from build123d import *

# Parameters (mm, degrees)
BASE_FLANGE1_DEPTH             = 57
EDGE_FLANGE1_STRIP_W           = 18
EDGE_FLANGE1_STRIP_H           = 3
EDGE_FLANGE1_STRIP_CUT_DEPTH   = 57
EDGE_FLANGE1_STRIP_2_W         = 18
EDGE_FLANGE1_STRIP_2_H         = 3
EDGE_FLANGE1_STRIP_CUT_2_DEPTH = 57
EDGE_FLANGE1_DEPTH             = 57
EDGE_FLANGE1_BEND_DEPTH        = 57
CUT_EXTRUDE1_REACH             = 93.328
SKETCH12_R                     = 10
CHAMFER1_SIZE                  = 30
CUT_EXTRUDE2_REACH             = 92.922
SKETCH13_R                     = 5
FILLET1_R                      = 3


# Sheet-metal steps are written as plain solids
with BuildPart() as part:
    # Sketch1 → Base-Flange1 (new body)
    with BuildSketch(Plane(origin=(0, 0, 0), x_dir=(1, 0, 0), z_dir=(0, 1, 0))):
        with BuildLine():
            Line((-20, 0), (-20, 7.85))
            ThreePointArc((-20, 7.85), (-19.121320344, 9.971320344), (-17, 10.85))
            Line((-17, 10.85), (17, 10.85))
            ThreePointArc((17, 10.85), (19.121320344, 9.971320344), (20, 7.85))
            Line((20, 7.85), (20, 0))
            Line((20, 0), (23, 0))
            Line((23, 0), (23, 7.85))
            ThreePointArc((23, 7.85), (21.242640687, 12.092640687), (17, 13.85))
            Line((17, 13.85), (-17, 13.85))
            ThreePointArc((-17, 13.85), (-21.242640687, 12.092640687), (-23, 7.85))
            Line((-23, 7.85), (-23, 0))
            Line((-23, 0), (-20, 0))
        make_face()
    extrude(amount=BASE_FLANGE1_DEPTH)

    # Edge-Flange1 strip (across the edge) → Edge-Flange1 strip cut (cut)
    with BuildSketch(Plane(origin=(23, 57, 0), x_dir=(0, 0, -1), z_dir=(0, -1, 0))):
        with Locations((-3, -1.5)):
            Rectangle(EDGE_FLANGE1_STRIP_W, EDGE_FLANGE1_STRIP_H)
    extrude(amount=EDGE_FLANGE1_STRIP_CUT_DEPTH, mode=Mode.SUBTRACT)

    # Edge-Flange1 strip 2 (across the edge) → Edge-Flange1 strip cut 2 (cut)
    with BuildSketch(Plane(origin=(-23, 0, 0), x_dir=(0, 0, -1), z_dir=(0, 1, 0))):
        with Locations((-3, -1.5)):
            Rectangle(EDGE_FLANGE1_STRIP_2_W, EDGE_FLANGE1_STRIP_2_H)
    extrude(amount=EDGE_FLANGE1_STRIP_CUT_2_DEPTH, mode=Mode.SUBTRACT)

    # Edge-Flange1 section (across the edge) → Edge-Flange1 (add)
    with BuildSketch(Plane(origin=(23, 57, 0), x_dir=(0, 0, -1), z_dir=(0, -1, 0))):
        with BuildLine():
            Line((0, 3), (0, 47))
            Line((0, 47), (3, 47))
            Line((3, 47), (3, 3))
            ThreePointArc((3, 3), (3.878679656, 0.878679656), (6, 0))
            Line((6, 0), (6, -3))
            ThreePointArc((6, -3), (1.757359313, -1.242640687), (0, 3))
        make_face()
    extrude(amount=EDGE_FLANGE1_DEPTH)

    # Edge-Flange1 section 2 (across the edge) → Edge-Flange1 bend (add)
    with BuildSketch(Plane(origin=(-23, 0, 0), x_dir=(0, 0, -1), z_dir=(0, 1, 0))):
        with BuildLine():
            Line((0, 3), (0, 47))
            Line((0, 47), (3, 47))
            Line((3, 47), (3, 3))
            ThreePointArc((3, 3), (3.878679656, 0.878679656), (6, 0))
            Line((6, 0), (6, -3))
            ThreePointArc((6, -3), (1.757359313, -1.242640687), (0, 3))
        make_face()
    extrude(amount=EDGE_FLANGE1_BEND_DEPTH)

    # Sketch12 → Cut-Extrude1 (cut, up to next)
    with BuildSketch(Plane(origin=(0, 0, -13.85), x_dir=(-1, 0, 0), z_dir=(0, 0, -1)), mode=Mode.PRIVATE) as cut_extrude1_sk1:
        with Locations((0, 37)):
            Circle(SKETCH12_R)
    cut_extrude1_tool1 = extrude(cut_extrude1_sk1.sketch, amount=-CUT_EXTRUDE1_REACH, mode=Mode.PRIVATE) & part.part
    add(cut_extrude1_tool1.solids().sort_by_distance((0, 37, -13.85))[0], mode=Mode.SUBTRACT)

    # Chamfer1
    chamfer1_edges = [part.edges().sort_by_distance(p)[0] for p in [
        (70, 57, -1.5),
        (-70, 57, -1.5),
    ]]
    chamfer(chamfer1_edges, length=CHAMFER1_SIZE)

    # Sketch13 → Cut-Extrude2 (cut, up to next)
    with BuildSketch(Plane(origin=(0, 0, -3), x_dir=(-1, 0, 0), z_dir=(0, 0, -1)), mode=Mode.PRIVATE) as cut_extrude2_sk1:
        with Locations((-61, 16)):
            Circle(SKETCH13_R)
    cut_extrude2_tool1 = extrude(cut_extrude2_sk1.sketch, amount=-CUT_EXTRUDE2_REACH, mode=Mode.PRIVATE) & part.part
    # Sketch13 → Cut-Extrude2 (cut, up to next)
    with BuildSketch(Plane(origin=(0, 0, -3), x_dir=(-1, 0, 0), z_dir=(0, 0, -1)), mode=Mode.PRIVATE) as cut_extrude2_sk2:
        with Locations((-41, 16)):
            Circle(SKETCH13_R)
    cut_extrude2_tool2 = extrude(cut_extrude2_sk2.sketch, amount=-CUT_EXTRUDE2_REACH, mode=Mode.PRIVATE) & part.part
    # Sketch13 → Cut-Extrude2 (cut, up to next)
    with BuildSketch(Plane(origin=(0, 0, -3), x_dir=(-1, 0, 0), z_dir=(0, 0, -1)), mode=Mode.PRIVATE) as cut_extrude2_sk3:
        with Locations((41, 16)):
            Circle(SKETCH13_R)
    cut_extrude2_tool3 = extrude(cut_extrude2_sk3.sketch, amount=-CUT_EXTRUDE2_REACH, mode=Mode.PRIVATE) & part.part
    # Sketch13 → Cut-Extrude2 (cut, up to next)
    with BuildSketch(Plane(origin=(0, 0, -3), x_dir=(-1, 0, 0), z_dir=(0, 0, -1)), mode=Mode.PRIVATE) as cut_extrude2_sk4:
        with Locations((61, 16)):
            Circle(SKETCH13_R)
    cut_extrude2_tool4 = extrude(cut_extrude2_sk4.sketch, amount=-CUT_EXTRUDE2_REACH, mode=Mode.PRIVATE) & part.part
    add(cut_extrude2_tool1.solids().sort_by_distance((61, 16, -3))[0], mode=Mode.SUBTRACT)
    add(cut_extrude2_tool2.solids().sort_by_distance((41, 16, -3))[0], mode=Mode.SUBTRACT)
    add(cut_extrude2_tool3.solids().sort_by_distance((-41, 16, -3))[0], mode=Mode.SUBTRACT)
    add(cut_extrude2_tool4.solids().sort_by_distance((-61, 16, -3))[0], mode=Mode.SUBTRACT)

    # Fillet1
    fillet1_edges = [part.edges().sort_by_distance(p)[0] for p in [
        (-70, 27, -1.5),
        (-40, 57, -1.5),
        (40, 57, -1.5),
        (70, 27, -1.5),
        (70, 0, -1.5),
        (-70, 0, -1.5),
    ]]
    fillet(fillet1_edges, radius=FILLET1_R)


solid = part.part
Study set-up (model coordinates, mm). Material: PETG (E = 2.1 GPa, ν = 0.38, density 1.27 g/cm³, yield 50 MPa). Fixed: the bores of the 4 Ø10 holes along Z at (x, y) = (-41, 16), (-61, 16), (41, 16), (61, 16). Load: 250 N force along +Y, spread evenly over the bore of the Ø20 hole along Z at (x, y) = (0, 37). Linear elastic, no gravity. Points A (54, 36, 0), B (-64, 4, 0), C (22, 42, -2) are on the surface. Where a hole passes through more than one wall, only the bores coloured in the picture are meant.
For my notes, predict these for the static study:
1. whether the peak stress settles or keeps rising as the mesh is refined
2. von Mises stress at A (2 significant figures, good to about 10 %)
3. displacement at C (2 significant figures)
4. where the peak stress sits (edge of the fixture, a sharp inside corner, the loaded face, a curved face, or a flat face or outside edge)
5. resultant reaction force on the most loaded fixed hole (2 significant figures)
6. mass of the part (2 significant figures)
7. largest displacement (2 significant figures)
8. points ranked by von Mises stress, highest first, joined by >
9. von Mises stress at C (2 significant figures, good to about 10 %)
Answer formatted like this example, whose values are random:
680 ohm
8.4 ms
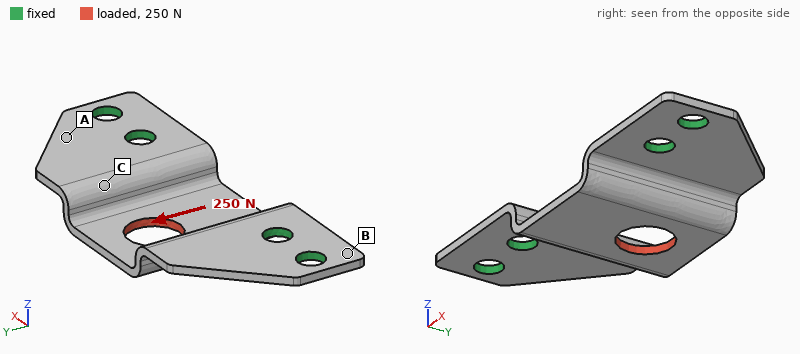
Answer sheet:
keeps rising
7.1 MPa
0.99 mm
edge of the fixture
220 N
28 g
1.7 mm
A > C > B
3.7 MPa
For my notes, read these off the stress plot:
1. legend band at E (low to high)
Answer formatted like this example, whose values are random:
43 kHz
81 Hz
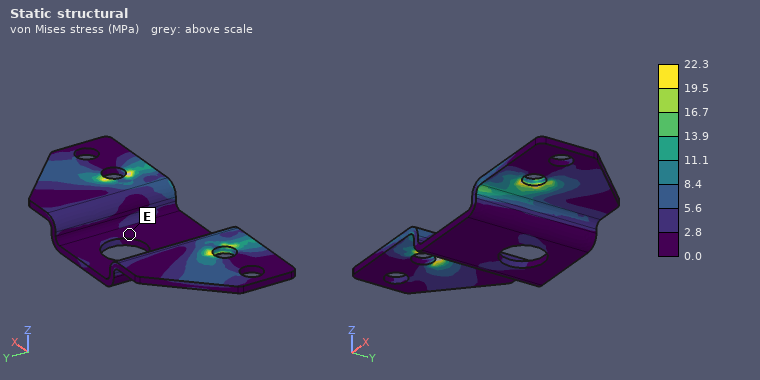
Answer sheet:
0.0 to 2.8 MPa
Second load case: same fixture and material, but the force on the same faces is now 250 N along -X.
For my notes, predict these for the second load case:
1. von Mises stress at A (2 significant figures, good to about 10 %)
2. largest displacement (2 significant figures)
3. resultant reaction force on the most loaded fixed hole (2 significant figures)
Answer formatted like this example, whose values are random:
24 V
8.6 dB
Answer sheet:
1.0 MPa
0.35 mm
100 N
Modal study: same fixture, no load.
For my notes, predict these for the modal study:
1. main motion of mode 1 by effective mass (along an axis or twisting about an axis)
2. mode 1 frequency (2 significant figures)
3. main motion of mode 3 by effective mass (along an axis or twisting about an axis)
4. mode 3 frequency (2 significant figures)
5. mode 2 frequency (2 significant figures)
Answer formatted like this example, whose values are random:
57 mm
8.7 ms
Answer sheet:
along Z
440 Hz
along Z
1300 Hz
890 Hz
